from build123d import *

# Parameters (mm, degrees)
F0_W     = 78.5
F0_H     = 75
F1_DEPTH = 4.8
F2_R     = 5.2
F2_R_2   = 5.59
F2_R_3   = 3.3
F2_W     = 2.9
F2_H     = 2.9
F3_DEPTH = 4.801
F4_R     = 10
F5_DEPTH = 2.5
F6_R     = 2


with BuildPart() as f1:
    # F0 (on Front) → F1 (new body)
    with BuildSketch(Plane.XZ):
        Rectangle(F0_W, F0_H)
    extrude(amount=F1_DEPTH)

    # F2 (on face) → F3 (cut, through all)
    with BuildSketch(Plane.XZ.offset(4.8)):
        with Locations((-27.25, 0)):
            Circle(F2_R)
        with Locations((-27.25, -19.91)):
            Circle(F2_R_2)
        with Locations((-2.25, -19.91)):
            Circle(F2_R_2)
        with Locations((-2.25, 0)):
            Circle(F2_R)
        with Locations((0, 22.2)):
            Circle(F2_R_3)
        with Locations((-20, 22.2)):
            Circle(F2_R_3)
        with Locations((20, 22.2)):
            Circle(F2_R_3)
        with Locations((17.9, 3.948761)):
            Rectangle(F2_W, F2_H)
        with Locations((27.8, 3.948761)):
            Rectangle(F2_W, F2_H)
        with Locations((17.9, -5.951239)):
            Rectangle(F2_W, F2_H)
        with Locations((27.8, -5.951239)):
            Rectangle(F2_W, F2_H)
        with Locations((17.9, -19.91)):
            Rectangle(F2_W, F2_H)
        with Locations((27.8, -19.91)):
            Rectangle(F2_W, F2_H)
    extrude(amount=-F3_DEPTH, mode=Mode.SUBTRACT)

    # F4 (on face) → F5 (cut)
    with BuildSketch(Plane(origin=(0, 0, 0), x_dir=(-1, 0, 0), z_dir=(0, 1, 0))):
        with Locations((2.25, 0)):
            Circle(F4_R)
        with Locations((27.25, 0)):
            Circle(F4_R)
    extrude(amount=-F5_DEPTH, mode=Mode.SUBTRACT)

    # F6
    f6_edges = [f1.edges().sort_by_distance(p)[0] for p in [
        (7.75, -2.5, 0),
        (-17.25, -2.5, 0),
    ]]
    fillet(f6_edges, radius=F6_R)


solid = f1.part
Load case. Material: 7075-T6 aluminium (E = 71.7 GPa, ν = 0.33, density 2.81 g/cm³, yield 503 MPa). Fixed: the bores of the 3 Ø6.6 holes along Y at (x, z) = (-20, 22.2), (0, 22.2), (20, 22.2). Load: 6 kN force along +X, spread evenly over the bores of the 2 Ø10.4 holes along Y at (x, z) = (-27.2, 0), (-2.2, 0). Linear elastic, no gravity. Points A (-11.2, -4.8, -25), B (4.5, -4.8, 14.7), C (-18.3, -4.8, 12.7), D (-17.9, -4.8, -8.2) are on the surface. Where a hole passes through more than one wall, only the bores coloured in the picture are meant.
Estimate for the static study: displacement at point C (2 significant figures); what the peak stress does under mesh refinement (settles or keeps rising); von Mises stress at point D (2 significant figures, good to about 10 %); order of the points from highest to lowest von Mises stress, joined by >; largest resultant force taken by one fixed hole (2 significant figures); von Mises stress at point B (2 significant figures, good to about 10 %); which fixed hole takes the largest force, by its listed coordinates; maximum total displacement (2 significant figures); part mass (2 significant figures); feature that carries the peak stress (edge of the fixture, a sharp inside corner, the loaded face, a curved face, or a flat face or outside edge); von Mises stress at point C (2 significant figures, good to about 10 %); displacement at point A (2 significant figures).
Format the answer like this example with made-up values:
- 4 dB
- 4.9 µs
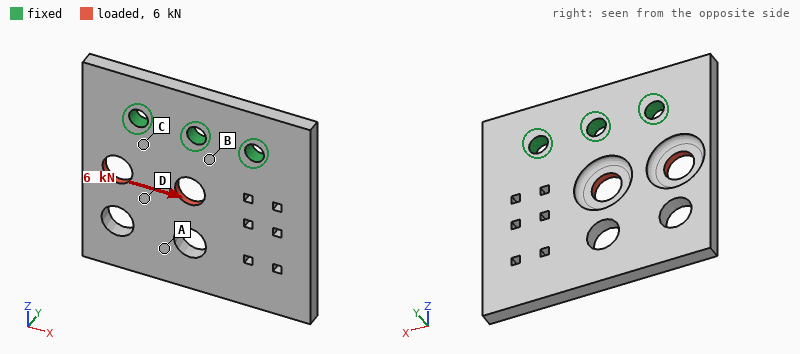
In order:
- 11 µm
- keeps rising
- 27 MPa
- C > B > D > A
- 3.8 kN
- 47 MPa
- (-20, 22.2)
- 70 µm
- 69 g
- edge of the fixture
- 65 MPa
- 45 µm
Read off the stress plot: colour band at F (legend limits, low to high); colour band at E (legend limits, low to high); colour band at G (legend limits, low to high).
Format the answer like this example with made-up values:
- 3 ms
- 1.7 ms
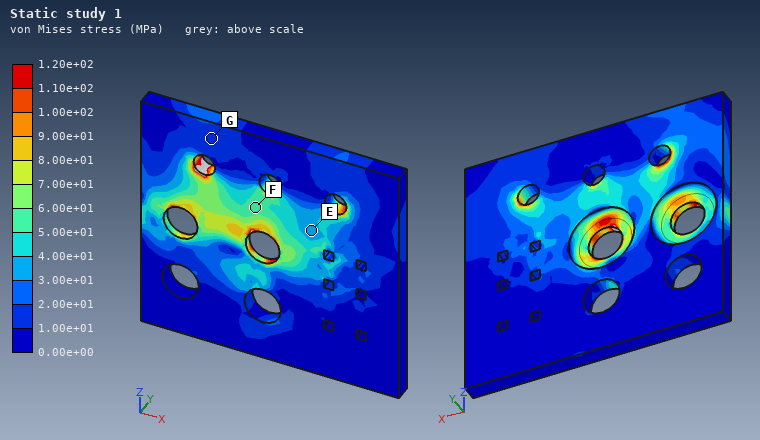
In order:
- 5.00e+01 to 6.00e+01 MPa
- 3.00e+01 to 4.00e+01 MPa
- 1.00e+01 to 2.00e+01 MPa
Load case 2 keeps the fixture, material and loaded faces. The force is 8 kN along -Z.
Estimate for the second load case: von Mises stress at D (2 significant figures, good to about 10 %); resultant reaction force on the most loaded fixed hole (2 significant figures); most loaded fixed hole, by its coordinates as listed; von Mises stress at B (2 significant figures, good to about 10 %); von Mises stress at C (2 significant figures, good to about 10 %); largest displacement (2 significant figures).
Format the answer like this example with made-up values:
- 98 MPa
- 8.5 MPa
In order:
- 36 MPa
- 5.6 kN
- (-20, 22.2)
- 54 MPa
- 95 MPa
- 0.25 mm
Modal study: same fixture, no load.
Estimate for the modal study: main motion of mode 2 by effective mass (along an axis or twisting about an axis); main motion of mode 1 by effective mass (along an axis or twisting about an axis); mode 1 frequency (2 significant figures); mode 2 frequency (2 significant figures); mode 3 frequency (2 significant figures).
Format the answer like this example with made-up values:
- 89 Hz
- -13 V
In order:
- twisting about Z
- along Y
- 1000 Hz
- 1900 Hz
- 4700 Hz
